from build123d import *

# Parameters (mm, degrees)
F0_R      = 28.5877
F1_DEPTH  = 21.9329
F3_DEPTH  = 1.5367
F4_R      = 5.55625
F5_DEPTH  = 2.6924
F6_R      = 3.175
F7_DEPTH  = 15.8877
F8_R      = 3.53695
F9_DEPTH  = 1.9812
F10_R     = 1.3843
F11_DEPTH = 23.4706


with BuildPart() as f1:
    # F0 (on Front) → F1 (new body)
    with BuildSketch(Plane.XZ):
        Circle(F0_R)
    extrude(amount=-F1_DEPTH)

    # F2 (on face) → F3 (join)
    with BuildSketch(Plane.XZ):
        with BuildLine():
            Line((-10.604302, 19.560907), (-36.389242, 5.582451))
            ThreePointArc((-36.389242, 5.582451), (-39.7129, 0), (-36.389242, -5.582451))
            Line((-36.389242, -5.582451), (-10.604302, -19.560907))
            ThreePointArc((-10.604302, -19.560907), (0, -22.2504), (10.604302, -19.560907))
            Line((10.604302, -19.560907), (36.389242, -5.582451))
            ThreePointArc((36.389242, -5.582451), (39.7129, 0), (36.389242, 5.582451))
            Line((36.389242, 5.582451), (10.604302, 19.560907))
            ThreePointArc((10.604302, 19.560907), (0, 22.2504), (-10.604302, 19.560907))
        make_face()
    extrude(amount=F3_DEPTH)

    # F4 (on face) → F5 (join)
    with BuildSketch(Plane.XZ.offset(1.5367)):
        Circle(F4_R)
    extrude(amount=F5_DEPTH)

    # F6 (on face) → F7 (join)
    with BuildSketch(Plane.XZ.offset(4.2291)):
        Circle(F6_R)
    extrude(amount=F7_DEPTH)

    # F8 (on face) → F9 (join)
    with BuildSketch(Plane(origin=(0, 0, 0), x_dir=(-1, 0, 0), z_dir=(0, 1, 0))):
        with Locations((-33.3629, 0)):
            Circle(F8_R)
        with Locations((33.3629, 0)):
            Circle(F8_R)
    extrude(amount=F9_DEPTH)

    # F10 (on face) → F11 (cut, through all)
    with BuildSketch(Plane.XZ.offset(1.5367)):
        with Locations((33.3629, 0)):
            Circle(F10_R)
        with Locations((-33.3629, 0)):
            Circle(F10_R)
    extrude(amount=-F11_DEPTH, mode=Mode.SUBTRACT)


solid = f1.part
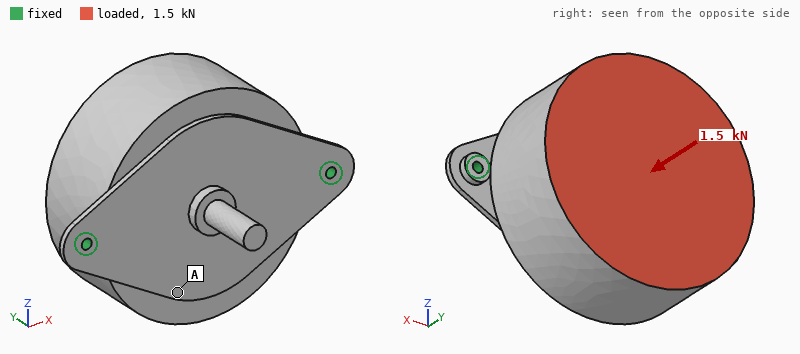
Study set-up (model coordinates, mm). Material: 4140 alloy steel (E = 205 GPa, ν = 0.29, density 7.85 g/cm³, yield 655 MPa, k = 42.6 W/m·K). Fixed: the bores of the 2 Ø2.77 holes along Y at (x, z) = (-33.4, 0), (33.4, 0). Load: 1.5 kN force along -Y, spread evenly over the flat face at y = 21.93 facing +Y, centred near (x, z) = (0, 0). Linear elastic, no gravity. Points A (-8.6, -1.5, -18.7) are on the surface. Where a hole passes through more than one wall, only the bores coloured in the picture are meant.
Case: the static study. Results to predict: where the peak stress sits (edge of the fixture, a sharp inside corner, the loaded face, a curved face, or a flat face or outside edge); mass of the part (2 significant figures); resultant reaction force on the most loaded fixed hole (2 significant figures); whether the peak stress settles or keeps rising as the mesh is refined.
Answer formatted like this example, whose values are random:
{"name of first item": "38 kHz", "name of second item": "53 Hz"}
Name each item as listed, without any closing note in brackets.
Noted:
{"where the peak stress sits": "edge of the fixture", "mass of the part": "480 g", "resultant reaction force on the most loaded fixed hole": "780 N", "whether the peak stress settles or keeps rising as the mesh is refined": "keeps rising"}
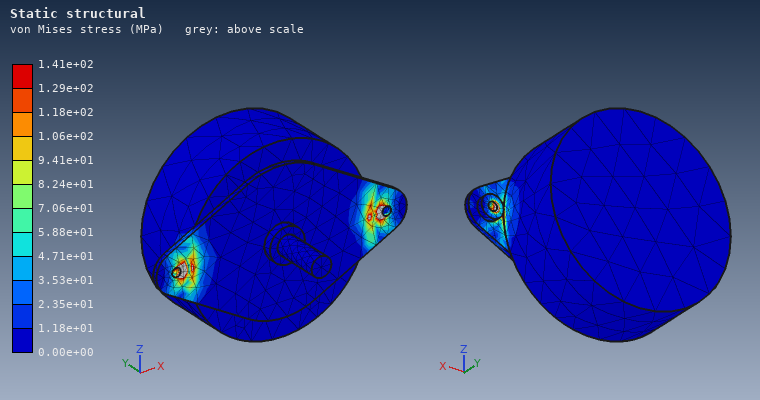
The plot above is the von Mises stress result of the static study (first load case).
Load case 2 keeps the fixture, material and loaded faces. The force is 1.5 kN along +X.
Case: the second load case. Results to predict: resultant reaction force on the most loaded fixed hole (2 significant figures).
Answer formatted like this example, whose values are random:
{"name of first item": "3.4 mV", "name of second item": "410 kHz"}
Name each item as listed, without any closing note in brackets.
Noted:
{"resultant reaction force on the most loaded fixed hole": "940 N"}
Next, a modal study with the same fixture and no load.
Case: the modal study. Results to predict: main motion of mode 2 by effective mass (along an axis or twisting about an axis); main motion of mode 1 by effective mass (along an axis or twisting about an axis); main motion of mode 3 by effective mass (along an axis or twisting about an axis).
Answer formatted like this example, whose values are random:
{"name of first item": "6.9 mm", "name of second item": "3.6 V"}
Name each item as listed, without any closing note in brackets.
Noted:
{"main motion of mode 2 by effective mass": "along Y", "main motion of mode 1 by effective mass": "along Z", "main motion of mode 3 by effective mass": "along X"}
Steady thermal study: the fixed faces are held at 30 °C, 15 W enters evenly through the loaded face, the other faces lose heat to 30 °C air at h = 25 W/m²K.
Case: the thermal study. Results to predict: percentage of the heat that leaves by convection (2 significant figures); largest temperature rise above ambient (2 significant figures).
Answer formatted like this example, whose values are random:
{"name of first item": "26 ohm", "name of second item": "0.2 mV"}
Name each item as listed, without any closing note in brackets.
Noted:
{"percentage of the heat that leaves by convection": "40 %", "largest temperature rise above ambient": "35 K"}
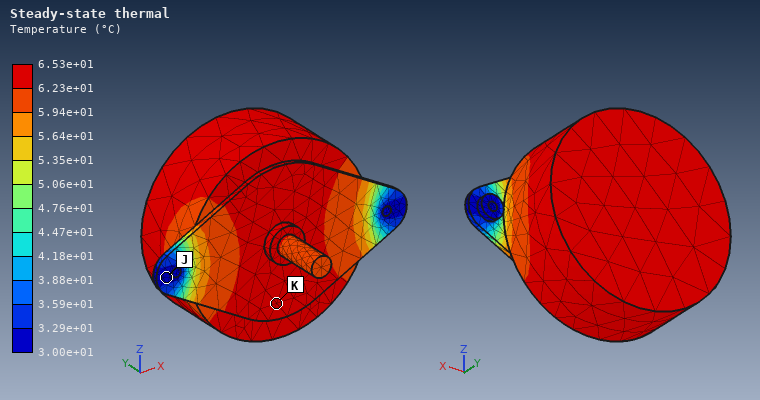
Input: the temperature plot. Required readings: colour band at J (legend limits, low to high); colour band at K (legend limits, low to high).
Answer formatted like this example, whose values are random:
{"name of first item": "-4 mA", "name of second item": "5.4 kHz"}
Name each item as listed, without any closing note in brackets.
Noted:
{"colour band at J": "3.00e+01 to 3.29e+01 °C", "colour band at K": "6.23e+01 to 6.53e+01 °C"}
